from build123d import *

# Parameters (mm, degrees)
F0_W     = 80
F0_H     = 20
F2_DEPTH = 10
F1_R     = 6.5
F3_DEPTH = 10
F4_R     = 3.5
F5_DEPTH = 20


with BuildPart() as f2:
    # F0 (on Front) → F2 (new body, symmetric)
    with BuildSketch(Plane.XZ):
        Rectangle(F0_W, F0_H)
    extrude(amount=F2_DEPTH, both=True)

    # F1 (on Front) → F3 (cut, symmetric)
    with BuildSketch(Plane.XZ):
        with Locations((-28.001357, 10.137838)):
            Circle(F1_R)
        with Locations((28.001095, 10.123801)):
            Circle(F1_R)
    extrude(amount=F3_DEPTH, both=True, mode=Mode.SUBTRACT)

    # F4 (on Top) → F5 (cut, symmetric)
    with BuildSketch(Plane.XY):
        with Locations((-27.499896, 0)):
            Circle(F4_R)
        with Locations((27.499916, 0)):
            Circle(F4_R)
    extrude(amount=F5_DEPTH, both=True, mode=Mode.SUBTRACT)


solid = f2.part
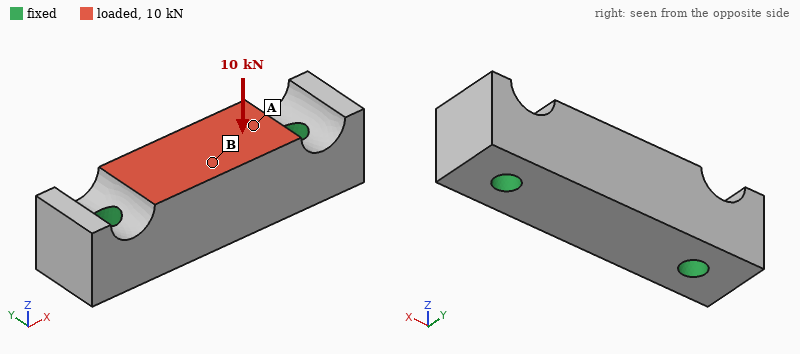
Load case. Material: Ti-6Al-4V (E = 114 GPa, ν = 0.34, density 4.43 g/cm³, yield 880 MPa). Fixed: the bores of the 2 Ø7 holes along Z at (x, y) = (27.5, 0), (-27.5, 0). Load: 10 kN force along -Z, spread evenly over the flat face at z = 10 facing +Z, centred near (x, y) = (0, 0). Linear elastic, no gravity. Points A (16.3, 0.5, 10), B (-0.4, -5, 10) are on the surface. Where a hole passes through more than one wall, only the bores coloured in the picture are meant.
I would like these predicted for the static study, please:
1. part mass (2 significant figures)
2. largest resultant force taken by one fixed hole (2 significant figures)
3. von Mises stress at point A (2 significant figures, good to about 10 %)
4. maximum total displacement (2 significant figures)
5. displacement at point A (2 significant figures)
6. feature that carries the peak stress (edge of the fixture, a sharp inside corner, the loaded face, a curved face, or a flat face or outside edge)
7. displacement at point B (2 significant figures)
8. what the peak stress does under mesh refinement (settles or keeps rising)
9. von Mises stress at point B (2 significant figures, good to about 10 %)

130 g
5.3 kN
16 MPa
11 µm
7.3 µm
edge of the fixture
11 µm
keeps rising
31 MPa
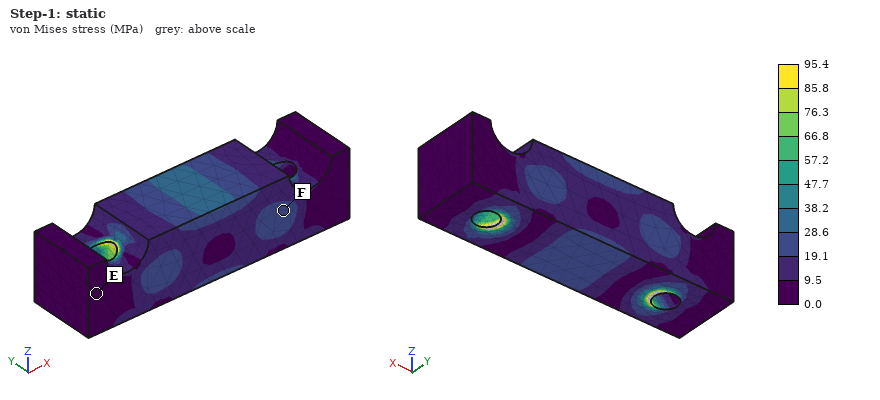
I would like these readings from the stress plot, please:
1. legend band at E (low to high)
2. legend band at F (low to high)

0.0 to 9.5 MPa
19.1 to 28.6 MPa
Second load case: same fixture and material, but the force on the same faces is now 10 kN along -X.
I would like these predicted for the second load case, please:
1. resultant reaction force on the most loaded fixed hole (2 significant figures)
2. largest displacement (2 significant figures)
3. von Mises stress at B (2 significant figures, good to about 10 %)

5.5 kN
4.6 µm
20 MPa
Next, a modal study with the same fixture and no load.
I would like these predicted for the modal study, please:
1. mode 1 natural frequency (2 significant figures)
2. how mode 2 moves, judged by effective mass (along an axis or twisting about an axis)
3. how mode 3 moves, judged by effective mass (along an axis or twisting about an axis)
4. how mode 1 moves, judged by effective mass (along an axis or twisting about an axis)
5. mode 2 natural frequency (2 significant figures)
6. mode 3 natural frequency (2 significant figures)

17 kHz
along Z
twisting about X
along Y
19 kHz
23 kHz
